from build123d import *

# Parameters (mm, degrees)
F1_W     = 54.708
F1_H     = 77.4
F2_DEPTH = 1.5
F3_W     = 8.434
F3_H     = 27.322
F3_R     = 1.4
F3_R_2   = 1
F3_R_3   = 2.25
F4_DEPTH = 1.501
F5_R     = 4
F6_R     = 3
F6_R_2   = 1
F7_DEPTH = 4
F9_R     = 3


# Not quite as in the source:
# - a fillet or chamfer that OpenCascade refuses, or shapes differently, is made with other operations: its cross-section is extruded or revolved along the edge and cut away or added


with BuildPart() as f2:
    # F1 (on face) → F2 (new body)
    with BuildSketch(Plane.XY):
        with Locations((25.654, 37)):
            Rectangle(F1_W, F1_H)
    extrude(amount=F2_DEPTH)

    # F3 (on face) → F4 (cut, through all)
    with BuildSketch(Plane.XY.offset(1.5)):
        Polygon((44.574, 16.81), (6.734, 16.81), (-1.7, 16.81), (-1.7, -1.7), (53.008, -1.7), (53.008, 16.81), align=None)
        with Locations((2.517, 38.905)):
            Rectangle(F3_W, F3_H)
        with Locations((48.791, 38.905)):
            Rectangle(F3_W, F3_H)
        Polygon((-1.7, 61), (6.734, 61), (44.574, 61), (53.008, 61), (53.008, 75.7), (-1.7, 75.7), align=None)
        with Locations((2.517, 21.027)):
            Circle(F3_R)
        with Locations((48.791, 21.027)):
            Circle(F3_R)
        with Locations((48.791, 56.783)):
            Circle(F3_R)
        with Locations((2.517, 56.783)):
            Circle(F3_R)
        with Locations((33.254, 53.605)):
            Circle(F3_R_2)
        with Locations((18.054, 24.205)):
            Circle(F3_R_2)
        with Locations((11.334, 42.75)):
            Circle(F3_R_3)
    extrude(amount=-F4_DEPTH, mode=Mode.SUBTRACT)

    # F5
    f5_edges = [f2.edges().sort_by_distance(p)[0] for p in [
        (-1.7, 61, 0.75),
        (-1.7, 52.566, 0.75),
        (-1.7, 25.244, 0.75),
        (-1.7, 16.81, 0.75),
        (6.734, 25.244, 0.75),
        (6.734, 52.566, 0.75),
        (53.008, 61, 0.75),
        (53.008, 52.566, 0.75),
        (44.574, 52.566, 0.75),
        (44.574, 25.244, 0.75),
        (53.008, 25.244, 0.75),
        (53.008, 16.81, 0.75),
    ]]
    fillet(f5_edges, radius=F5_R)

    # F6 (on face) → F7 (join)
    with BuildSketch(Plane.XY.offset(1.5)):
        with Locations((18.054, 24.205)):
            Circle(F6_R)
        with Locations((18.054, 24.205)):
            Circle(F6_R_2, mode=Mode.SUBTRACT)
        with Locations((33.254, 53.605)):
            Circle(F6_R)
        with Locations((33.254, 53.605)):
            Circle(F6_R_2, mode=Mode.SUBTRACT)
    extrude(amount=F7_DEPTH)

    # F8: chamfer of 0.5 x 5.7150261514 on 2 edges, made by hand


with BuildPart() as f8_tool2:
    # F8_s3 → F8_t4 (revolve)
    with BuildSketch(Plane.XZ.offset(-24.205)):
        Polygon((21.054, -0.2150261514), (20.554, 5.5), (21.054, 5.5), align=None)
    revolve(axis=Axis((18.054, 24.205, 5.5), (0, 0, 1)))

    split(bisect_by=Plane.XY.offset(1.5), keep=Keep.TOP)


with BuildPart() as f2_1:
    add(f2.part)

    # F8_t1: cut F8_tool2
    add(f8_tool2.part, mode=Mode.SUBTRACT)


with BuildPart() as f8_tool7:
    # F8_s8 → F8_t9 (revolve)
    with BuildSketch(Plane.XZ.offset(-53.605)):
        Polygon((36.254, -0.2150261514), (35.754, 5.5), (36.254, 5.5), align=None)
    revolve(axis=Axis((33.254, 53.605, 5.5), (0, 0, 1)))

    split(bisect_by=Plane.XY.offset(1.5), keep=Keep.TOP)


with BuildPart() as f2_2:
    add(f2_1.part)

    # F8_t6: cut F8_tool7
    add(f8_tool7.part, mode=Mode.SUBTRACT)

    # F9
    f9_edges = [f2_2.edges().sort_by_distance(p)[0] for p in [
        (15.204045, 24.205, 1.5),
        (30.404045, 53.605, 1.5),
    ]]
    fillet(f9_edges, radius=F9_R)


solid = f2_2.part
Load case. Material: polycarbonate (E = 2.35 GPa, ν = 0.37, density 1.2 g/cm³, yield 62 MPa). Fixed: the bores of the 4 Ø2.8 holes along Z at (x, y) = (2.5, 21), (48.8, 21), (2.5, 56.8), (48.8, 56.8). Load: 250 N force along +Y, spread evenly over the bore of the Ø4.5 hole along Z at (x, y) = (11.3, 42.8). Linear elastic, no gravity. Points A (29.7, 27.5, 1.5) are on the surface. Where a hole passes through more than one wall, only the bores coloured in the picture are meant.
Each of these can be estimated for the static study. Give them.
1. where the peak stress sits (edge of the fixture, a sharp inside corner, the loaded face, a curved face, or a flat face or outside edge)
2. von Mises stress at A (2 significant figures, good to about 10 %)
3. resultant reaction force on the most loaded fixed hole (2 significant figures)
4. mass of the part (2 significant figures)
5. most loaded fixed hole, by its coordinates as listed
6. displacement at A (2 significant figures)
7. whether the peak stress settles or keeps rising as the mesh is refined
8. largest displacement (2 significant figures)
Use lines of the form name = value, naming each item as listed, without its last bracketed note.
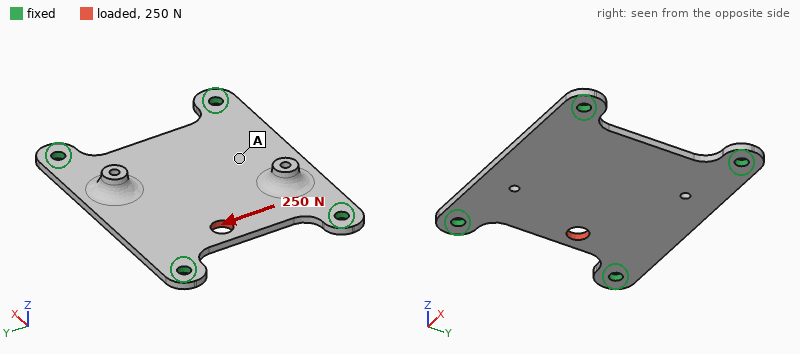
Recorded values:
where the peak stress sits = edge of the fixture
von Mises stress at A = 3.1 MPa
resultant reaction force on the most loaded fixed hole = 99 N
mass of the part = 3.7 g
most loaded fixed hole, by its coordinates as listed = (2.5, 56.8)
displacement at A = 0.059 mm
whether the peak stress settles or keeps rising as the mesh is refined = keeps rising
largest displacement = 0.12 mm
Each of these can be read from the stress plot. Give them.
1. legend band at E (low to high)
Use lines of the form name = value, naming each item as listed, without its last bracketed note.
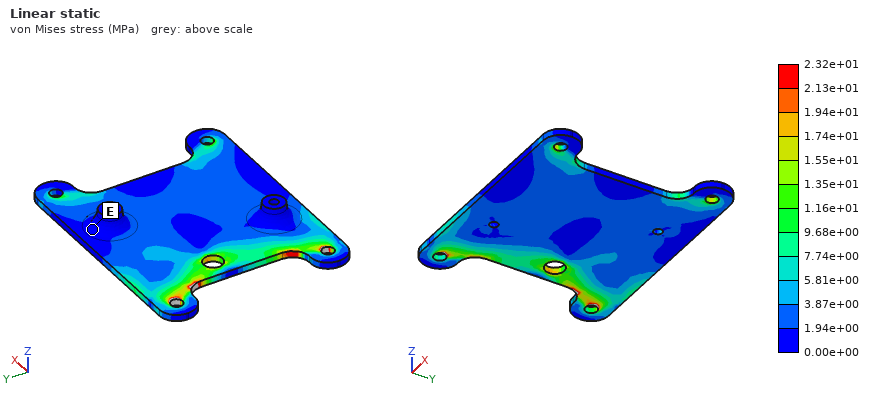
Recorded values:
legend band at E = 0.00e+00 to 1.94e+00 MPa
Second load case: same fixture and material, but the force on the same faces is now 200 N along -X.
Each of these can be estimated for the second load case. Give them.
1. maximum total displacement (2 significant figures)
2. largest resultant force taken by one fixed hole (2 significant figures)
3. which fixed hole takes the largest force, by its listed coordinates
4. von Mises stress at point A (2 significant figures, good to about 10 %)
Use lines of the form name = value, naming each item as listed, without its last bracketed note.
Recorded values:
maximum total displacement = 0.11 mm
largest resultant force taken by one fixed hole = 74 N
which fixed hole takes the largest force, by its listed coordinates = (2.5, 56.8)
von Mises stress at point A = 2.3 MPa
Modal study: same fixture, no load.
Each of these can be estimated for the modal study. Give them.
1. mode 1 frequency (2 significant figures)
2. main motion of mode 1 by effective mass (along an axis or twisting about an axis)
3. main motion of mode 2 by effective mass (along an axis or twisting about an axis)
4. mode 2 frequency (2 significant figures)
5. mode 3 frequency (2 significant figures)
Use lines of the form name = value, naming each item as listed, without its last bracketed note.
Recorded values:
mode 1 frequency = 790 Hz
main motion of mode 1 by effective mass = along Z
main motion of mode 2 by effective mass = twisting about X
mode 2 frequency = 1200 Hz
mode 3 frequency = 1700 Hz
